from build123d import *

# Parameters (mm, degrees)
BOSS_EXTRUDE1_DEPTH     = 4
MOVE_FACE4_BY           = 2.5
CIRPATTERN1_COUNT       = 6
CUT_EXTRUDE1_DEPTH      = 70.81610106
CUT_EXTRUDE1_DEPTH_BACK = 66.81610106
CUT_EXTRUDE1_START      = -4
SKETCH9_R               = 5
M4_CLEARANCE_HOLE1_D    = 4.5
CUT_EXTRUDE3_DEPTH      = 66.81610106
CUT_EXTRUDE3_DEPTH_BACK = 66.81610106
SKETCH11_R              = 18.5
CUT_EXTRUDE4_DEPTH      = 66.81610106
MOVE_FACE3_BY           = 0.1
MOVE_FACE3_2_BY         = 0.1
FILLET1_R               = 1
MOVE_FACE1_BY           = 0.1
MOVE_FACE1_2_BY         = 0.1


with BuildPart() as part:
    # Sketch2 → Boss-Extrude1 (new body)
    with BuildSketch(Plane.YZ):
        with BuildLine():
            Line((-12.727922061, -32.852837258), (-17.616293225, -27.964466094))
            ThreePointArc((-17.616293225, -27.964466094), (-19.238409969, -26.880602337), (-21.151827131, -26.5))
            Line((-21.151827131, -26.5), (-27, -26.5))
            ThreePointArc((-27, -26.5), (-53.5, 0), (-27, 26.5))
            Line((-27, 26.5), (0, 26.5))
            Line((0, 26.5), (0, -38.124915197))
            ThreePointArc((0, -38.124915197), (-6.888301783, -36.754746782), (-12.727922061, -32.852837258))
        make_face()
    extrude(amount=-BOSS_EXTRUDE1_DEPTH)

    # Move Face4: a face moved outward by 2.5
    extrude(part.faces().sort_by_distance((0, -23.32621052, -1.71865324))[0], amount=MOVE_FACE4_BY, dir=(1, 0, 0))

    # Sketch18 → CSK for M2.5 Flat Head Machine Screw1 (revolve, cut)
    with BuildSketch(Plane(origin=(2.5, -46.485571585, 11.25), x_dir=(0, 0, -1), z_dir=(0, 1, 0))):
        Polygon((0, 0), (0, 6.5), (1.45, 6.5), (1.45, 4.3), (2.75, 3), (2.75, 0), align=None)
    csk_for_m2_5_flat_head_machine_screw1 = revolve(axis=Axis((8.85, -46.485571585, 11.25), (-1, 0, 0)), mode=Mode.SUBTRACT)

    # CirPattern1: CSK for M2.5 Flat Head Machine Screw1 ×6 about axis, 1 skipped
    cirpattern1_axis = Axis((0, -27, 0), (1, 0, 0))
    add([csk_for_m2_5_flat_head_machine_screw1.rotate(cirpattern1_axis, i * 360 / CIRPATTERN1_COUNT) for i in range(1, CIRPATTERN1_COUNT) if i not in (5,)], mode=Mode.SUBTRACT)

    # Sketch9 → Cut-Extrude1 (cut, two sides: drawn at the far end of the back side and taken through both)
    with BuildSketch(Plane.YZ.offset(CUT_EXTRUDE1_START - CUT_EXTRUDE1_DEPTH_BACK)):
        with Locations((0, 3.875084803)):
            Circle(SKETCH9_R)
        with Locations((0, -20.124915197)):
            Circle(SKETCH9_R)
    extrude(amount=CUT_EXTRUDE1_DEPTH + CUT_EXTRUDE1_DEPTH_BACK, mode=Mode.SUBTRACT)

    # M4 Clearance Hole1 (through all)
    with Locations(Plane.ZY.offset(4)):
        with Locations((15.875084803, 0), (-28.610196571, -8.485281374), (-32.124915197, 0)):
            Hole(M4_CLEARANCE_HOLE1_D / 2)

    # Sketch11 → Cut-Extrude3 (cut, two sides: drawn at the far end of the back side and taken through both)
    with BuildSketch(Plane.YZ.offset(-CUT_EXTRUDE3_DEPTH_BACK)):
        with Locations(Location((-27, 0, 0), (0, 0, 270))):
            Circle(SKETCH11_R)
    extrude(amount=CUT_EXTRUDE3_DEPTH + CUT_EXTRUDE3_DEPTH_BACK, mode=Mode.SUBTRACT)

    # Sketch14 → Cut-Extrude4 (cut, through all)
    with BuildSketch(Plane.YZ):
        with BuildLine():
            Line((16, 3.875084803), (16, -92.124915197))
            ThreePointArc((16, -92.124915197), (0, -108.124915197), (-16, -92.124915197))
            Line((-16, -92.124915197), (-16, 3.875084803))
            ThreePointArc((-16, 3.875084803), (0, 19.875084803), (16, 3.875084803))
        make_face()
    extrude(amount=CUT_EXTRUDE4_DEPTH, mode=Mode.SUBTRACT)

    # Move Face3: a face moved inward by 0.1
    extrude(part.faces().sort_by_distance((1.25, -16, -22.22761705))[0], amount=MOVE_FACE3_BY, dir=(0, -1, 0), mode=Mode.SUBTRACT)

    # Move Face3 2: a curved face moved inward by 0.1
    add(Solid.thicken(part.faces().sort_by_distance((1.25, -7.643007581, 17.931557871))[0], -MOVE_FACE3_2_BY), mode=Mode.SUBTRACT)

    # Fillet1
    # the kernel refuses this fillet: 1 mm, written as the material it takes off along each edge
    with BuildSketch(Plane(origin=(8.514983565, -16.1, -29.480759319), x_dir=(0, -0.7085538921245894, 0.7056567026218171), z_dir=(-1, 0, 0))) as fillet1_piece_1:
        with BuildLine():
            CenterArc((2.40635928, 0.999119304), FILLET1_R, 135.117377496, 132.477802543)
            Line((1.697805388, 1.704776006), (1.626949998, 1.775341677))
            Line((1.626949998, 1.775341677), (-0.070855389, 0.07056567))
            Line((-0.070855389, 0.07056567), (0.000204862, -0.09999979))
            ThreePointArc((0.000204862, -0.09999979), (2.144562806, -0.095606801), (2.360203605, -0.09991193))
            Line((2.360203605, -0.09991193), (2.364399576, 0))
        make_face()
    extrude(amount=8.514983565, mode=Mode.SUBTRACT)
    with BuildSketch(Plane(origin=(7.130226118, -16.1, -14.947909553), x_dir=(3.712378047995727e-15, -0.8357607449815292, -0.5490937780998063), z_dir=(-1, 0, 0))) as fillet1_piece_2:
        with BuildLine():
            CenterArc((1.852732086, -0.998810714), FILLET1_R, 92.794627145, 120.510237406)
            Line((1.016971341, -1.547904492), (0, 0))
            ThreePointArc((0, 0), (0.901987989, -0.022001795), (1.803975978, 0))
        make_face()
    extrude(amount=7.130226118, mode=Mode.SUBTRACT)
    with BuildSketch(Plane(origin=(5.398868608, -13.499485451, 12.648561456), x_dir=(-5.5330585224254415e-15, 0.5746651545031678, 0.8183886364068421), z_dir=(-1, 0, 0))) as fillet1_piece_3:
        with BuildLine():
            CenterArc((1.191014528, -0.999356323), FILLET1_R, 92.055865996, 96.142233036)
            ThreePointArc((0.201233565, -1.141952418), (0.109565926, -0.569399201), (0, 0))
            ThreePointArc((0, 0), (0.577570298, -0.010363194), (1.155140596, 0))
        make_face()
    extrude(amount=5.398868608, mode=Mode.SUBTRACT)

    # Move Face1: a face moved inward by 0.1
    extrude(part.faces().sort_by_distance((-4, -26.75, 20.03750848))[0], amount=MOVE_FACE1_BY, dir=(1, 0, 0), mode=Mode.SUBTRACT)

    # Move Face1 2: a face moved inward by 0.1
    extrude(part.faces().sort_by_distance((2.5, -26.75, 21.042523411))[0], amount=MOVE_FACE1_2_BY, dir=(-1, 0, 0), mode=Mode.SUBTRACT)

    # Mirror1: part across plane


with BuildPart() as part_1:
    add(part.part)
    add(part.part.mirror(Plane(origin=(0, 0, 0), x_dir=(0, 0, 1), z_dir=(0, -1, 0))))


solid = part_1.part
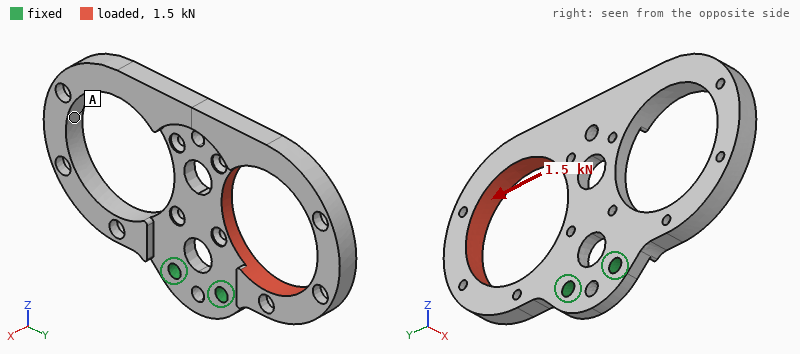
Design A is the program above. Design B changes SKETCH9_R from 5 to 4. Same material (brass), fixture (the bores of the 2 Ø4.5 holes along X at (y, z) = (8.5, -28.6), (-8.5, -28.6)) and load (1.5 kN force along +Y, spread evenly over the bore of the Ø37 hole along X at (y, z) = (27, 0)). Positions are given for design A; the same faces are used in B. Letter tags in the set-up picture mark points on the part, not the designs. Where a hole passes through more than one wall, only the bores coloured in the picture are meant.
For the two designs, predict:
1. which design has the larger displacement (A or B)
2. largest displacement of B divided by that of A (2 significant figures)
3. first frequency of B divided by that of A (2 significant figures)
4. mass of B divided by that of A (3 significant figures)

A
0.91
1.0
1.01
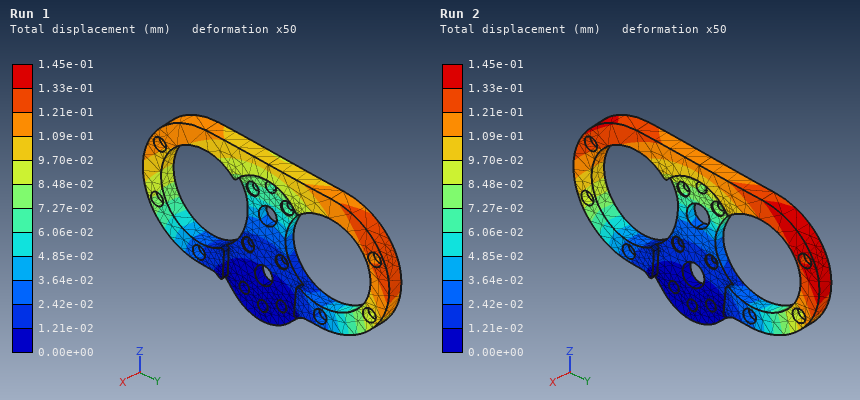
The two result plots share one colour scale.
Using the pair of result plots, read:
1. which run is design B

Run 1
